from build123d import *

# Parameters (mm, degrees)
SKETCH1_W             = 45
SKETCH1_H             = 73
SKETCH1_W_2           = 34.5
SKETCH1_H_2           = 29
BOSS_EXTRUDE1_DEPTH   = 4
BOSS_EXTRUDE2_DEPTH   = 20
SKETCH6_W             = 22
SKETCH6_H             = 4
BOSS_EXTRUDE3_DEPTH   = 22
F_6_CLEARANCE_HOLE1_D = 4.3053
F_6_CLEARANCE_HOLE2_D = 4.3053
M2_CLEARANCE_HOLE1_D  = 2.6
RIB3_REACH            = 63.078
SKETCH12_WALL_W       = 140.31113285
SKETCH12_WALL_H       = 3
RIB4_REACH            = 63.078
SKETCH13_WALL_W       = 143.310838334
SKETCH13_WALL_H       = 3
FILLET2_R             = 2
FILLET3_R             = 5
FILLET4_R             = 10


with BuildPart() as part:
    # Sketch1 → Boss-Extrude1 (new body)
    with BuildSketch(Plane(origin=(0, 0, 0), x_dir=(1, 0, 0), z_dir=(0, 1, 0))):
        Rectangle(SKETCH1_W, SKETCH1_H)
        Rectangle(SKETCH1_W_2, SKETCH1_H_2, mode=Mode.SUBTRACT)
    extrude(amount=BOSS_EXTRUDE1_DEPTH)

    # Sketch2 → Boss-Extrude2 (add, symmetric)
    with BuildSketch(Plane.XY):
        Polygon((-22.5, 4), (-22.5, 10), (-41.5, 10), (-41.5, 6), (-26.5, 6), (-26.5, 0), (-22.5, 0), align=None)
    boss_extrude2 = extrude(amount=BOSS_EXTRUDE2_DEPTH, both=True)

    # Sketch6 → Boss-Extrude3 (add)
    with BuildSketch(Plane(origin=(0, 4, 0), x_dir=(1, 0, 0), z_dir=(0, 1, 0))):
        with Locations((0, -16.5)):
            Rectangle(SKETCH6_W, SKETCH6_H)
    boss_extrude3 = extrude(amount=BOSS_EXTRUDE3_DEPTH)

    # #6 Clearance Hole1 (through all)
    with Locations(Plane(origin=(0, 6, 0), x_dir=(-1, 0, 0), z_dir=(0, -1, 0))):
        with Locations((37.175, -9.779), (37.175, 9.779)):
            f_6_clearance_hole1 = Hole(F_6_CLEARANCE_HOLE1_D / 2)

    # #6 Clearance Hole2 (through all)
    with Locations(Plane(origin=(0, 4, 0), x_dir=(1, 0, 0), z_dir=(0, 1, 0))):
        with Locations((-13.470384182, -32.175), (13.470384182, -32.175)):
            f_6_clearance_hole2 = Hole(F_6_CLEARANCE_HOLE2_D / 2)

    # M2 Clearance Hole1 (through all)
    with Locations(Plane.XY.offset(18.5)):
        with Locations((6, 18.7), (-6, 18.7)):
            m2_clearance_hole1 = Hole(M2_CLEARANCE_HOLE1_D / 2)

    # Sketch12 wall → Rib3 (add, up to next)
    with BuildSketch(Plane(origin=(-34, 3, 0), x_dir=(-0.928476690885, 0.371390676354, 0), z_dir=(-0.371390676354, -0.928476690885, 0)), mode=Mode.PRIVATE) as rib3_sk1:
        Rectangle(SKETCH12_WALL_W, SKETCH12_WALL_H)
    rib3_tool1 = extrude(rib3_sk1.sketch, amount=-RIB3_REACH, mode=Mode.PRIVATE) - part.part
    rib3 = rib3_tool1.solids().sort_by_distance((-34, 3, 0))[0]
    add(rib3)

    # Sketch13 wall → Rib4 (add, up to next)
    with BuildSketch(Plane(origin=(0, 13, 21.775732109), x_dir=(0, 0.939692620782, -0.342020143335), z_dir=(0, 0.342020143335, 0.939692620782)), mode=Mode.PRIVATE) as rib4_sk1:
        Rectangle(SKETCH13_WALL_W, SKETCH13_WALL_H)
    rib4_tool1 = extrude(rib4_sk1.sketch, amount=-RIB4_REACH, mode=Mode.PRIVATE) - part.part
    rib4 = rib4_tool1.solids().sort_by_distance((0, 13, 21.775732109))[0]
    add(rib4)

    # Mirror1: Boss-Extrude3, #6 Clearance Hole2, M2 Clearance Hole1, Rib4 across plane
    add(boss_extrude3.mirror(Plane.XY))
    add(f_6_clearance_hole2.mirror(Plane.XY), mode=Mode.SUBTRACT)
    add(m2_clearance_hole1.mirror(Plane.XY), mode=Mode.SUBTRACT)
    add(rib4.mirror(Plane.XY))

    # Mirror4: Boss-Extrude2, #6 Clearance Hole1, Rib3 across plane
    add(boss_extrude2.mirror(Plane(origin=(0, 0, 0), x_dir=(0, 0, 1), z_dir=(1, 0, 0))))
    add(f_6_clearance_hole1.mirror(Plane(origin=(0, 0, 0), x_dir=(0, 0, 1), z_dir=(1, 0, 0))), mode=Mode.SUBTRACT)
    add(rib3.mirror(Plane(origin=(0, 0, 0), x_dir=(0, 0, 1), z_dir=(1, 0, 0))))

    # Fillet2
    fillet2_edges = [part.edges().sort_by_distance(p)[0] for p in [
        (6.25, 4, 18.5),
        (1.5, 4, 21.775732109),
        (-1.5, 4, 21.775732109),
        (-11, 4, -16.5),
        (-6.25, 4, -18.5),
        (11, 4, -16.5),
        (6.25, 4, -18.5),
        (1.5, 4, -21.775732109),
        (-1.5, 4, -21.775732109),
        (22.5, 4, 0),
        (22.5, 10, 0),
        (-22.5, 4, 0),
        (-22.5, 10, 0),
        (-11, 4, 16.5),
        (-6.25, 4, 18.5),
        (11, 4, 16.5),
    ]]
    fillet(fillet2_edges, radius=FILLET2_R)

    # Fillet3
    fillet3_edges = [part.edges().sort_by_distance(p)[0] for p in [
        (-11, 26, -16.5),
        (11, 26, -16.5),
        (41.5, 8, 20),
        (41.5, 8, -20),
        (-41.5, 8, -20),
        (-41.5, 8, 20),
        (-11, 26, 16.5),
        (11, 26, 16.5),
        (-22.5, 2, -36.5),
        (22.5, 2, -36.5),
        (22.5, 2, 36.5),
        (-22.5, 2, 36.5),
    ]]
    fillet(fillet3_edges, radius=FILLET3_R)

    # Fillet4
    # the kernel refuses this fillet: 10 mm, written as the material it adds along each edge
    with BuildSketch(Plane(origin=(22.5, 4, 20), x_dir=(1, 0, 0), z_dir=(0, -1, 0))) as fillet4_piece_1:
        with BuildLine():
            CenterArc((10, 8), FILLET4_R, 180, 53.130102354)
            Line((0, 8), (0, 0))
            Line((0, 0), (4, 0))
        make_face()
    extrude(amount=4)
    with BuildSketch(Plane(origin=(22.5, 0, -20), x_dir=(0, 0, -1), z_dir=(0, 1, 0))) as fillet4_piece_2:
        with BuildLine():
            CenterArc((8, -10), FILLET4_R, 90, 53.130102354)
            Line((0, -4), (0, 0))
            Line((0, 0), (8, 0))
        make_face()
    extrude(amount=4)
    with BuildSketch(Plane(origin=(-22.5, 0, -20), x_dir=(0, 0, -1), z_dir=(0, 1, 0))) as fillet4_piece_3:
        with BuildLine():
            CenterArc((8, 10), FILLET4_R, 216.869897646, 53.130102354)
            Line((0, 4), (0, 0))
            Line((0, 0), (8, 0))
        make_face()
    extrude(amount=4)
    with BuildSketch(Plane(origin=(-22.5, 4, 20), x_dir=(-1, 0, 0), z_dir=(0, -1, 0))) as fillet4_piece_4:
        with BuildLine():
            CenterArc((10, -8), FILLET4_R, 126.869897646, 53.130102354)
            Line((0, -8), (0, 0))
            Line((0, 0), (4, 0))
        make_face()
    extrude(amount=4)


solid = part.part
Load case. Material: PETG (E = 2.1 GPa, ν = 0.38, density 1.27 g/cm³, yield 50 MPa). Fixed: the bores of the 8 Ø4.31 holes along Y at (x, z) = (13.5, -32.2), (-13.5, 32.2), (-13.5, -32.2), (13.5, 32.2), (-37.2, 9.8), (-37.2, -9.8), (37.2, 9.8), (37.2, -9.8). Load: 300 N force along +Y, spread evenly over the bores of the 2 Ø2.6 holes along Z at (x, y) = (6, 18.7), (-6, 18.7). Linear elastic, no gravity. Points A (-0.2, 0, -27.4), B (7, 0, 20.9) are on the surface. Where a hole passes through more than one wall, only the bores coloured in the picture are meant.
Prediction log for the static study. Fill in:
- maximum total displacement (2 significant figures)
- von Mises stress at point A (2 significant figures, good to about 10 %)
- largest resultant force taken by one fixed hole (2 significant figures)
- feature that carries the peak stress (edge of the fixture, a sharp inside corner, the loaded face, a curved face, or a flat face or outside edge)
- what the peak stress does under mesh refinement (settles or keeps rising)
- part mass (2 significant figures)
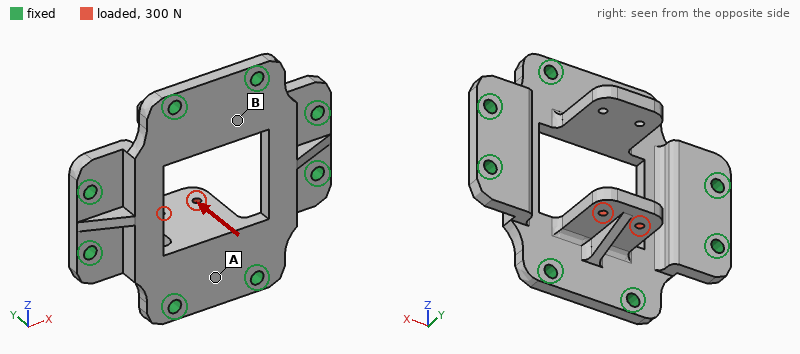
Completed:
1.0 mm
7.4 MPa
110 N
edge of the fixture
keeps rising
27 g
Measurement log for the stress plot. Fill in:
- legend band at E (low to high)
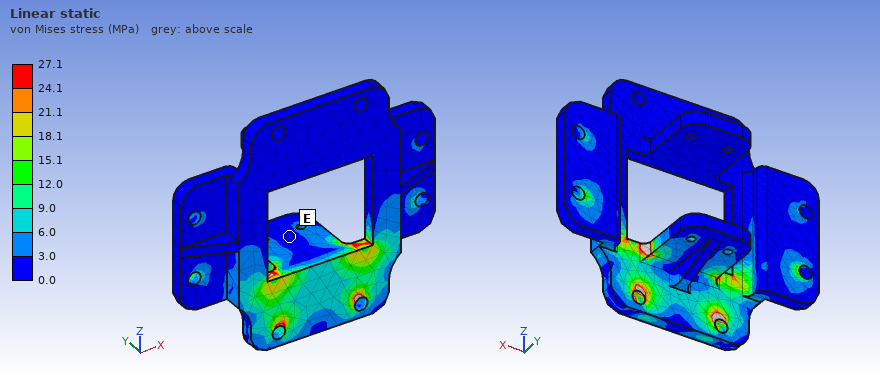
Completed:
0.0 to 3.0 MPa
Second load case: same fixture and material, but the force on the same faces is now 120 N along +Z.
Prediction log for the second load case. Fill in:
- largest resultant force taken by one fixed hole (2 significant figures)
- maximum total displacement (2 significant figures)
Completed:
99 N
1.1 mm
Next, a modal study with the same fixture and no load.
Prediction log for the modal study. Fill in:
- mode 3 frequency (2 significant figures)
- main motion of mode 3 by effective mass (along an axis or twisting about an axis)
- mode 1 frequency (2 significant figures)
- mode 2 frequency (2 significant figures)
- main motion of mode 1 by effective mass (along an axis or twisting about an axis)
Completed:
2300 Hz
along X
1300 Hz
1400 Hz
along Y
